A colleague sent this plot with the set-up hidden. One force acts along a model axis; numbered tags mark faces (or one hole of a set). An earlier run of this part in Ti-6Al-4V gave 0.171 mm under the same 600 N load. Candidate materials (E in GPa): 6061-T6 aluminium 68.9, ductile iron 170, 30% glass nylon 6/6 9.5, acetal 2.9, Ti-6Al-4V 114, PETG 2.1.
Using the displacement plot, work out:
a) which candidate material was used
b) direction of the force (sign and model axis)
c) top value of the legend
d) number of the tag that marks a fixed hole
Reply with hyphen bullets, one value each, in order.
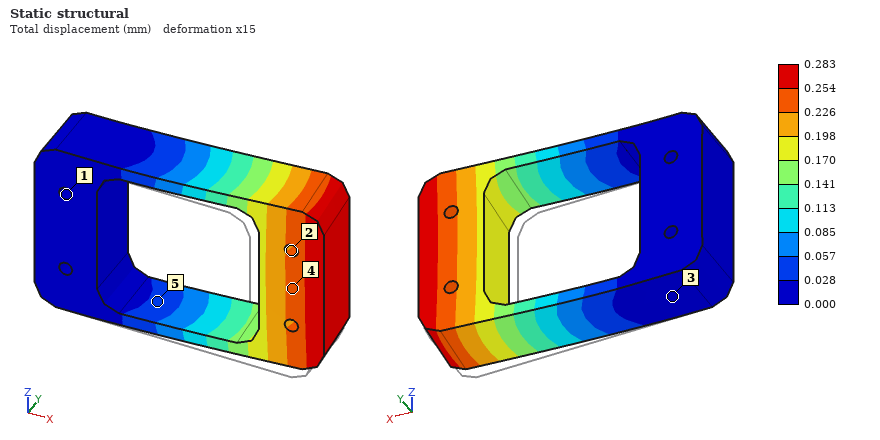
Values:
- 6061-T6 aluminium
- +Y
- 0.283 mm
- 1
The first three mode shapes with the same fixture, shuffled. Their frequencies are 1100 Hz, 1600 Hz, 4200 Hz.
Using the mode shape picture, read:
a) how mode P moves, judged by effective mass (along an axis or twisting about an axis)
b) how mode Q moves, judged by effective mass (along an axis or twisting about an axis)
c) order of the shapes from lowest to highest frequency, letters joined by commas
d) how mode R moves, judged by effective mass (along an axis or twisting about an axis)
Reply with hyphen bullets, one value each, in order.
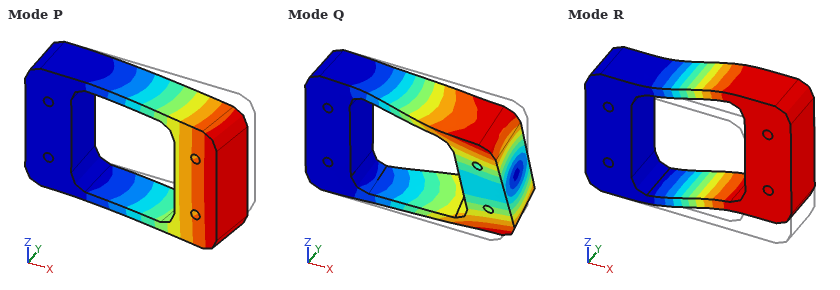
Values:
- along Y
- twisting about X
- R, P, Q
- along Z
